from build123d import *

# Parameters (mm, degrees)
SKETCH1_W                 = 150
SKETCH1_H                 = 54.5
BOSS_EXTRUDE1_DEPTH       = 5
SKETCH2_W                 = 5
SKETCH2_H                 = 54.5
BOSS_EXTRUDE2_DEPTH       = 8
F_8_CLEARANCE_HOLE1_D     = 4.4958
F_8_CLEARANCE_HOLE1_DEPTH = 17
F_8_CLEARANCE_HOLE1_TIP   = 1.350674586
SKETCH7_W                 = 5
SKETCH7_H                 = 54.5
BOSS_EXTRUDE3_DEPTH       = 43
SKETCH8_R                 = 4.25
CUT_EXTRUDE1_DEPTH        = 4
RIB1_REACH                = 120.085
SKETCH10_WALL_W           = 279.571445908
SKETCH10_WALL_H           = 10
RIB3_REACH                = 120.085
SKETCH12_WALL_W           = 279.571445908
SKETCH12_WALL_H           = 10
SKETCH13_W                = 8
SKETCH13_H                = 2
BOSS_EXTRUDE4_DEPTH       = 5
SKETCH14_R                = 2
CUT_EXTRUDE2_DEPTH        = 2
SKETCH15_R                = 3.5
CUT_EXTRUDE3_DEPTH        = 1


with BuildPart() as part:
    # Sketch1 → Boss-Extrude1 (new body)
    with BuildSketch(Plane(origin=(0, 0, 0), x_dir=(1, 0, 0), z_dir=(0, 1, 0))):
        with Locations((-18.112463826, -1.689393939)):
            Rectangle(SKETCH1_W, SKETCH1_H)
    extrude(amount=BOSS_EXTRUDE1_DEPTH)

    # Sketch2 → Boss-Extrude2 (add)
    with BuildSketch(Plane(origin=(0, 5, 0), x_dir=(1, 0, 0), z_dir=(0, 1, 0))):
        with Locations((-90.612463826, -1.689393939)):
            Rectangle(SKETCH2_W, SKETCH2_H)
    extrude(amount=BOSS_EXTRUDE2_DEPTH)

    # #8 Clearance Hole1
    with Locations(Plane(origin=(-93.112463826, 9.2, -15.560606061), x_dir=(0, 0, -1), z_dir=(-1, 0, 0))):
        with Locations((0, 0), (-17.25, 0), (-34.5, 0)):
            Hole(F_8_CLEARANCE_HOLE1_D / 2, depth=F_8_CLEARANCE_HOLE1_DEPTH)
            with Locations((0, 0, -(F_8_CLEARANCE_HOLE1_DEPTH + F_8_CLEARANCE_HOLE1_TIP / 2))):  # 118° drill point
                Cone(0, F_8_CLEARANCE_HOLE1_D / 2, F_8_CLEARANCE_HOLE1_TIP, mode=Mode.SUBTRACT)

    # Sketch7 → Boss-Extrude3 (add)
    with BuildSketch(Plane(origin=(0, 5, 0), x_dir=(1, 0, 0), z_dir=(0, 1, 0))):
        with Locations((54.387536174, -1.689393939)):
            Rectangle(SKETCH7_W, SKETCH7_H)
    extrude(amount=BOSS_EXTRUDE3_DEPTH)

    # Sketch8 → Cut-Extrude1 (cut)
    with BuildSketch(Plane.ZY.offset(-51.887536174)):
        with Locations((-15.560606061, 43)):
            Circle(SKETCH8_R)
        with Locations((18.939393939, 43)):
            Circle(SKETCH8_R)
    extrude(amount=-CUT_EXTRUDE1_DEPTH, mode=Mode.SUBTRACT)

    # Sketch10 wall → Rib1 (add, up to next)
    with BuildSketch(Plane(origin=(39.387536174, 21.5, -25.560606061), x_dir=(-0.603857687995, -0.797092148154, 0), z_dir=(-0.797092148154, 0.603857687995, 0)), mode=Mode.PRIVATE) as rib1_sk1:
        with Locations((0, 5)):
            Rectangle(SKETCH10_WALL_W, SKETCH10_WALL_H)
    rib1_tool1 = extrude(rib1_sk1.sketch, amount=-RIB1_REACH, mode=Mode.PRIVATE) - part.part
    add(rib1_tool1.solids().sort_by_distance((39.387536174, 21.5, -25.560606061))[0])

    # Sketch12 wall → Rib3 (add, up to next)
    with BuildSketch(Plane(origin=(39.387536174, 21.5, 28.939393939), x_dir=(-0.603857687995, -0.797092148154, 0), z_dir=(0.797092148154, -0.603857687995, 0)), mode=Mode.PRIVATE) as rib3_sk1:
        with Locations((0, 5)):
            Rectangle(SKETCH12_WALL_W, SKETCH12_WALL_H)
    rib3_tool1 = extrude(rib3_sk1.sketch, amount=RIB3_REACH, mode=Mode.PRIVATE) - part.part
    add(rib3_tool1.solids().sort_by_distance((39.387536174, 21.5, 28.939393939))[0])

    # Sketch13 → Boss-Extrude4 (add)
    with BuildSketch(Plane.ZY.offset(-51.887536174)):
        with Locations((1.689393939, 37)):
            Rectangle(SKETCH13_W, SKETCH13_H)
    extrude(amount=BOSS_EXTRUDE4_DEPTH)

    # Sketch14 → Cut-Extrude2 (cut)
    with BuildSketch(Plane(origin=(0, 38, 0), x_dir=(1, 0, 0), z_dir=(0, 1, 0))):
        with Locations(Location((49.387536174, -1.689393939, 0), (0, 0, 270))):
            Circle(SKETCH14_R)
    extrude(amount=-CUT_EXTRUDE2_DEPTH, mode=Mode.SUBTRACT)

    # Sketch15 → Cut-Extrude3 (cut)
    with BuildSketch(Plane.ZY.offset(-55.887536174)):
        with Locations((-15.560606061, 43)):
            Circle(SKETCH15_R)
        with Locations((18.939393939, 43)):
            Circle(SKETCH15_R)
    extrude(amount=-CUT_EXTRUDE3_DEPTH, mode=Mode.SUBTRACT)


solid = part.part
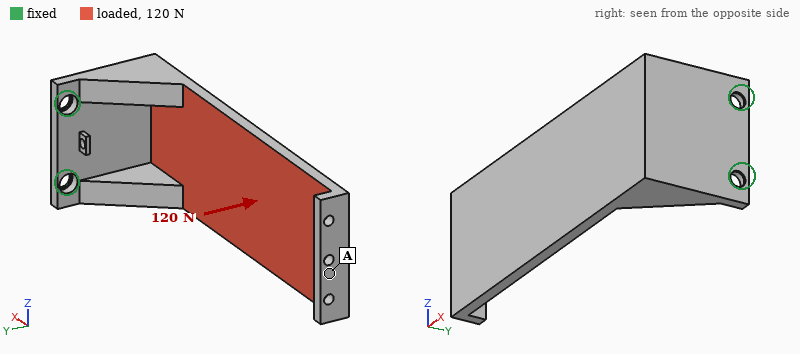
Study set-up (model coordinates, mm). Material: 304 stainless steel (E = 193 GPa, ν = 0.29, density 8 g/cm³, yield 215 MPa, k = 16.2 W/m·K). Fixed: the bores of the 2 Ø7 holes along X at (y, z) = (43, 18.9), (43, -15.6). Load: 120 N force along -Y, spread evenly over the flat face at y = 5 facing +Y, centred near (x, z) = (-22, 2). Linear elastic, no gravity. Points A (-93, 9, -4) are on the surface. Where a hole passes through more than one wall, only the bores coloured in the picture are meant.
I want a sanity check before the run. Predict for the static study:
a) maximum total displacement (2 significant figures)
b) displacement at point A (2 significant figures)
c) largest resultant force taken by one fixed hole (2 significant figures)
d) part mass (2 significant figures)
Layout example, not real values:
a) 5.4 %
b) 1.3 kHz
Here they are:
a) 0.58 mm
b) 0.58 mm
c) 120 N
d) 500 g
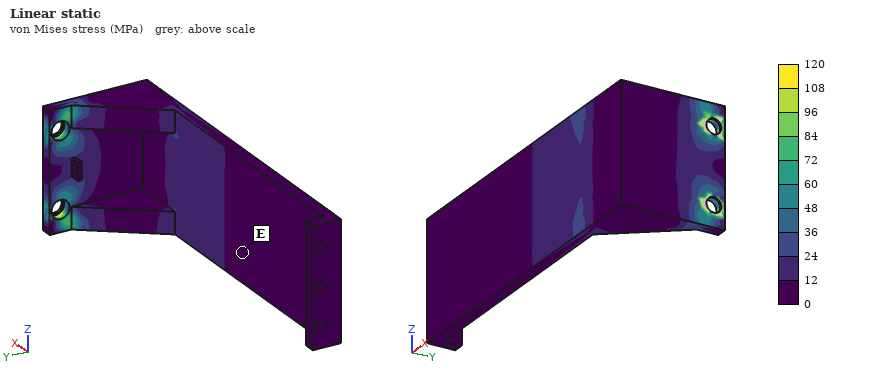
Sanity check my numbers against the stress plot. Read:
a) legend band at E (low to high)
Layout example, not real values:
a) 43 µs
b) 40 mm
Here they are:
a) 0 to 12 MPa
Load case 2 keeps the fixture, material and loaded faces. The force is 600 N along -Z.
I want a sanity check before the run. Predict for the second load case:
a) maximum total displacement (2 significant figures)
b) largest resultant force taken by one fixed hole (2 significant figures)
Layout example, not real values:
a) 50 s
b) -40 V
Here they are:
a) 0.44 mm
b) 1.4 kN
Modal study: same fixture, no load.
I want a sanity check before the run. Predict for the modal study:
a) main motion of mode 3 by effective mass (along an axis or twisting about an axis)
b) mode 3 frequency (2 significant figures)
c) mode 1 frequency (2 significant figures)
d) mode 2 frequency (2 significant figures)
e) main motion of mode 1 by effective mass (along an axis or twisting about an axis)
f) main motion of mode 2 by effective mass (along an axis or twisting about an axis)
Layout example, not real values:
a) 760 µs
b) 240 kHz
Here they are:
a) along X
b) 570 Hz
c) 140 Hz
d) 390 Hz
e) along Y
f) along Z
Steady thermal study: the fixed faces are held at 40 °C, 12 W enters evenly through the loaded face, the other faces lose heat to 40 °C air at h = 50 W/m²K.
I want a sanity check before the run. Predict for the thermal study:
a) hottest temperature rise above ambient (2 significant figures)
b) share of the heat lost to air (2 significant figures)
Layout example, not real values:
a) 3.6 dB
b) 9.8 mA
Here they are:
a) 23 K
b) 95 %
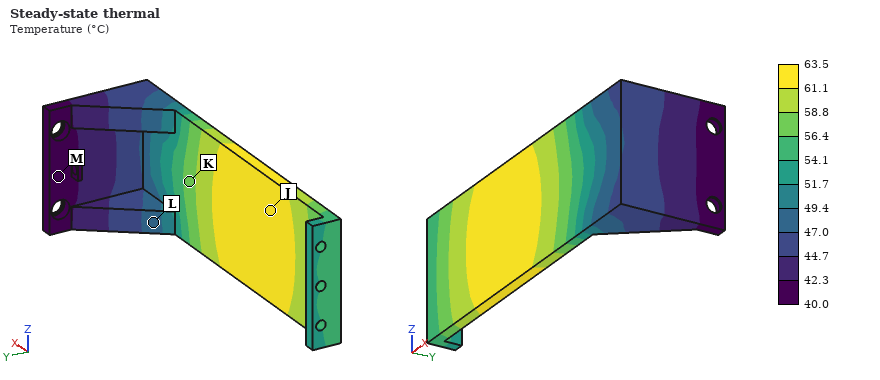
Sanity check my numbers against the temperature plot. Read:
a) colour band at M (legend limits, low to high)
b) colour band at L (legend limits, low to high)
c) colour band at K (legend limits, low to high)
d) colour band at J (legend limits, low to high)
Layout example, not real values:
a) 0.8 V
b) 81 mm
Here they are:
a) 40.0 to 42.3 °C
b) 47.0 to 49.4 °C
c) 56.4 to 58.8 °C
d) 61.1 to 63.5 °C
